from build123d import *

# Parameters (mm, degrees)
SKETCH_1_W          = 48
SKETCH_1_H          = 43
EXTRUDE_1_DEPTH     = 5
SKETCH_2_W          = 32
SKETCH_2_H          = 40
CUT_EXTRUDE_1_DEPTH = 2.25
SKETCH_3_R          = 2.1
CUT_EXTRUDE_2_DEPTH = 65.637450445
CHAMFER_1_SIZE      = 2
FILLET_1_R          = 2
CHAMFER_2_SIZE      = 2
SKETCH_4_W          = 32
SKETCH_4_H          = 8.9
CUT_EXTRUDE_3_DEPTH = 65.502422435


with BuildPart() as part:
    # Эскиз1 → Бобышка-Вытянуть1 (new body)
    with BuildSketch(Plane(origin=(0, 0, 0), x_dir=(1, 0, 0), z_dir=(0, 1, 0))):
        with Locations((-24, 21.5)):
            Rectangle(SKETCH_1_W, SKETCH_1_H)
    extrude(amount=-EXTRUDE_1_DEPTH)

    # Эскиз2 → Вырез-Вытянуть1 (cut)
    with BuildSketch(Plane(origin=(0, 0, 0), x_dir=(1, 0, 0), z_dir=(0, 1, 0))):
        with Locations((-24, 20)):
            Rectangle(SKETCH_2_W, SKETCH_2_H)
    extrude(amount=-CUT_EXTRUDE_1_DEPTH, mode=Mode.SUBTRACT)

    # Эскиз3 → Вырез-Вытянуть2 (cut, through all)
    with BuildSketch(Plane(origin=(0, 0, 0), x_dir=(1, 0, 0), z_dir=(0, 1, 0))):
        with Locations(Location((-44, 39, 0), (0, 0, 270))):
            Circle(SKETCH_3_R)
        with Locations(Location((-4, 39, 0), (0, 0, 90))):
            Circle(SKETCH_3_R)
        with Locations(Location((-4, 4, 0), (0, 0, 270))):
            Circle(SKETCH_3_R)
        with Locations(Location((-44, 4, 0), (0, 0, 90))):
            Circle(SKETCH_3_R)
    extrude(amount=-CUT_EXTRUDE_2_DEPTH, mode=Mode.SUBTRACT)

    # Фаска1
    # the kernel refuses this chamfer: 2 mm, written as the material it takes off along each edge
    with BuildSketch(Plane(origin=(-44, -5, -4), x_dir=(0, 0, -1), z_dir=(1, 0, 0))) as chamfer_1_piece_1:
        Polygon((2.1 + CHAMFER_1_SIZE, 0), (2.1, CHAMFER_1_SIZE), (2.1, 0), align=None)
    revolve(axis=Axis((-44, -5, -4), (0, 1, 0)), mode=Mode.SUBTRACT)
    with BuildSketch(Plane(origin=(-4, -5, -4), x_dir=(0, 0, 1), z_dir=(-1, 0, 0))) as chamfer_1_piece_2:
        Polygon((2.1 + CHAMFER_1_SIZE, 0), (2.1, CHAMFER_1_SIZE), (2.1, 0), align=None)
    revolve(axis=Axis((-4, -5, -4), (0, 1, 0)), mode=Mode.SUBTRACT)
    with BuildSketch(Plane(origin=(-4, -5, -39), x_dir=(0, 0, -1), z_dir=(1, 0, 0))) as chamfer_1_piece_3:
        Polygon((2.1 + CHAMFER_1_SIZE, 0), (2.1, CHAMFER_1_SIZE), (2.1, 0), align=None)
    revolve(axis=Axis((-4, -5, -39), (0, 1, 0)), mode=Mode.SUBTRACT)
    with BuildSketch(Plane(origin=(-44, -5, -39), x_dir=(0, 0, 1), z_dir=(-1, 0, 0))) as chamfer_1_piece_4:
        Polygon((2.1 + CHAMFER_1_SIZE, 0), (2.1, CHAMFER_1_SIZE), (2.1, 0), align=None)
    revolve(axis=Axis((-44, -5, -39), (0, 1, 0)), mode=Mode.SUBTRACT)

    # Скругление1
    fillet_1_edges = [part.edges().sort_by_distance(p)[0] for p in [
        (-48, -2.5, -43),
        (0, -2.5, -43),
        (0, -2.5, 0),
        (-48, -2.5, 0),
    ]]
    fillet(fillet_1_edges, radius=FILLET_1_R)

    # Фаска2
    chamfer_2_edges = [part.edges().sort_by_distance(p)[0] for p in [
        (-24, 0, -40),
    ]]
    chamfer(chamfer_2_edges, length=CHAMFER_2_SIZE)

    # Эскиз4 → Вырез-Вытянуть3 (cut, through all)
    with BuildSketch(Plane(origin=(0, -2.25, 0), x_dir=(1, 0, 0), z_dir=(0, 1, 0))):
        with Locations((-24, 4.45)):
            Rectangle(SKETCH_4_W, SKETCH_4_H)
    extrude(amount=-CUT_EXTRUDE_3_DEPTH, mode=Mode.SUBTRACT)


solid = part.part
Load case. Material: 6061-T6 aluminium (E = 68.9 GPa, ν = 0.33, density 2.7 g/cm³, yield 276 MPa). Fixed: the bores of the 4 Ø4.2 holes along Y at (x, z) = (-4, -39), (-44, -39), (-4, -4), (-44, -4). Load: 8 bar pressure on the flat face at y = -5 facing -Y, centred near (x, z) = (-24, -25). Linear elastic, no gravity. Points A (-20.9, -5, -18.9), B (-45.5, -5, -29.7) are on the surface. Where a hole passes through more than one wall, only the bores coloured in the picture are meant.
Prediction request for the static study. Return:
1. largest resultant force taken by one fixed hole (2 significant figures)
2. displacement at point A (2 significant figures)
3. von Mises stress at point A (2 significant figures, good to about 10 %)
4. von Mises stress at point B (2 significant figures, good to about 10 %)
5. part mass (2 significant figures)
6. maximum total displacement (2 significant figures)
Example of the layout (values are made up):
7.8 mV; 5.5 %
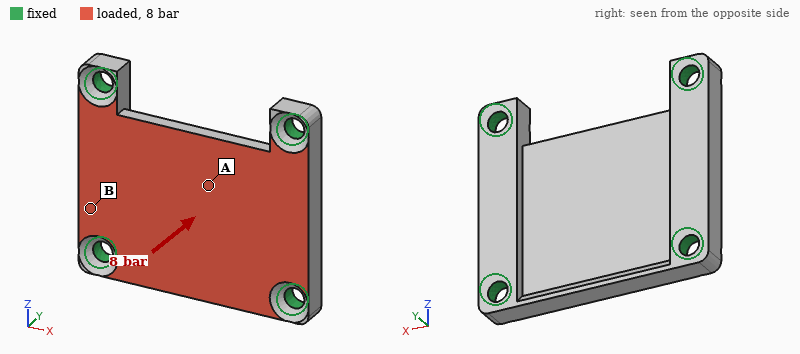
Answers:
520 N; 49 µm; 37 MPa; 14 MPa; 17 g; 53 µm
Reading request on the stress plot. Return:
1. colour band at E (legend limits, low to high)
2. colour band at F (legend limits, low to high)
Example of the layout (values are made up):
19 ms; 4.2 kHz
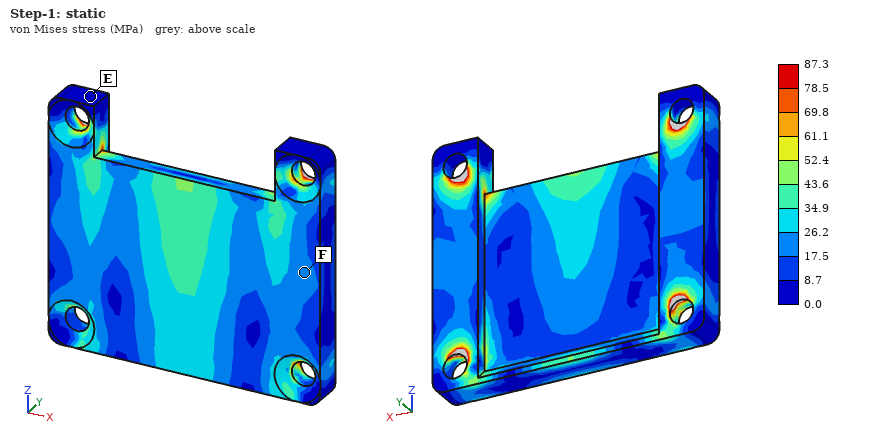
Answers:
0.0 to 8.7 MPa; 17.5 to 26.2 MPa
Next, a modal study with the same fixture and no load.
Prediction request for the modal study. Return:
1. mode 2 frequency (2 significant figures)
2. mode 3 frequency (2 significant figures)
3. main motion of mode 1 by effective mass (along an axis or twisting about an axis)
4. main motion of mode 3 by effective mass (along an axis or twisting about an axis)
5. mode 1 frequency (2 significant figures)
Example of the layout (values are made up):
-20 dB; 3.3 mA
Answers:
13 kHz; 16 kHz; along Y; twisting about Z; 8700 Hz
